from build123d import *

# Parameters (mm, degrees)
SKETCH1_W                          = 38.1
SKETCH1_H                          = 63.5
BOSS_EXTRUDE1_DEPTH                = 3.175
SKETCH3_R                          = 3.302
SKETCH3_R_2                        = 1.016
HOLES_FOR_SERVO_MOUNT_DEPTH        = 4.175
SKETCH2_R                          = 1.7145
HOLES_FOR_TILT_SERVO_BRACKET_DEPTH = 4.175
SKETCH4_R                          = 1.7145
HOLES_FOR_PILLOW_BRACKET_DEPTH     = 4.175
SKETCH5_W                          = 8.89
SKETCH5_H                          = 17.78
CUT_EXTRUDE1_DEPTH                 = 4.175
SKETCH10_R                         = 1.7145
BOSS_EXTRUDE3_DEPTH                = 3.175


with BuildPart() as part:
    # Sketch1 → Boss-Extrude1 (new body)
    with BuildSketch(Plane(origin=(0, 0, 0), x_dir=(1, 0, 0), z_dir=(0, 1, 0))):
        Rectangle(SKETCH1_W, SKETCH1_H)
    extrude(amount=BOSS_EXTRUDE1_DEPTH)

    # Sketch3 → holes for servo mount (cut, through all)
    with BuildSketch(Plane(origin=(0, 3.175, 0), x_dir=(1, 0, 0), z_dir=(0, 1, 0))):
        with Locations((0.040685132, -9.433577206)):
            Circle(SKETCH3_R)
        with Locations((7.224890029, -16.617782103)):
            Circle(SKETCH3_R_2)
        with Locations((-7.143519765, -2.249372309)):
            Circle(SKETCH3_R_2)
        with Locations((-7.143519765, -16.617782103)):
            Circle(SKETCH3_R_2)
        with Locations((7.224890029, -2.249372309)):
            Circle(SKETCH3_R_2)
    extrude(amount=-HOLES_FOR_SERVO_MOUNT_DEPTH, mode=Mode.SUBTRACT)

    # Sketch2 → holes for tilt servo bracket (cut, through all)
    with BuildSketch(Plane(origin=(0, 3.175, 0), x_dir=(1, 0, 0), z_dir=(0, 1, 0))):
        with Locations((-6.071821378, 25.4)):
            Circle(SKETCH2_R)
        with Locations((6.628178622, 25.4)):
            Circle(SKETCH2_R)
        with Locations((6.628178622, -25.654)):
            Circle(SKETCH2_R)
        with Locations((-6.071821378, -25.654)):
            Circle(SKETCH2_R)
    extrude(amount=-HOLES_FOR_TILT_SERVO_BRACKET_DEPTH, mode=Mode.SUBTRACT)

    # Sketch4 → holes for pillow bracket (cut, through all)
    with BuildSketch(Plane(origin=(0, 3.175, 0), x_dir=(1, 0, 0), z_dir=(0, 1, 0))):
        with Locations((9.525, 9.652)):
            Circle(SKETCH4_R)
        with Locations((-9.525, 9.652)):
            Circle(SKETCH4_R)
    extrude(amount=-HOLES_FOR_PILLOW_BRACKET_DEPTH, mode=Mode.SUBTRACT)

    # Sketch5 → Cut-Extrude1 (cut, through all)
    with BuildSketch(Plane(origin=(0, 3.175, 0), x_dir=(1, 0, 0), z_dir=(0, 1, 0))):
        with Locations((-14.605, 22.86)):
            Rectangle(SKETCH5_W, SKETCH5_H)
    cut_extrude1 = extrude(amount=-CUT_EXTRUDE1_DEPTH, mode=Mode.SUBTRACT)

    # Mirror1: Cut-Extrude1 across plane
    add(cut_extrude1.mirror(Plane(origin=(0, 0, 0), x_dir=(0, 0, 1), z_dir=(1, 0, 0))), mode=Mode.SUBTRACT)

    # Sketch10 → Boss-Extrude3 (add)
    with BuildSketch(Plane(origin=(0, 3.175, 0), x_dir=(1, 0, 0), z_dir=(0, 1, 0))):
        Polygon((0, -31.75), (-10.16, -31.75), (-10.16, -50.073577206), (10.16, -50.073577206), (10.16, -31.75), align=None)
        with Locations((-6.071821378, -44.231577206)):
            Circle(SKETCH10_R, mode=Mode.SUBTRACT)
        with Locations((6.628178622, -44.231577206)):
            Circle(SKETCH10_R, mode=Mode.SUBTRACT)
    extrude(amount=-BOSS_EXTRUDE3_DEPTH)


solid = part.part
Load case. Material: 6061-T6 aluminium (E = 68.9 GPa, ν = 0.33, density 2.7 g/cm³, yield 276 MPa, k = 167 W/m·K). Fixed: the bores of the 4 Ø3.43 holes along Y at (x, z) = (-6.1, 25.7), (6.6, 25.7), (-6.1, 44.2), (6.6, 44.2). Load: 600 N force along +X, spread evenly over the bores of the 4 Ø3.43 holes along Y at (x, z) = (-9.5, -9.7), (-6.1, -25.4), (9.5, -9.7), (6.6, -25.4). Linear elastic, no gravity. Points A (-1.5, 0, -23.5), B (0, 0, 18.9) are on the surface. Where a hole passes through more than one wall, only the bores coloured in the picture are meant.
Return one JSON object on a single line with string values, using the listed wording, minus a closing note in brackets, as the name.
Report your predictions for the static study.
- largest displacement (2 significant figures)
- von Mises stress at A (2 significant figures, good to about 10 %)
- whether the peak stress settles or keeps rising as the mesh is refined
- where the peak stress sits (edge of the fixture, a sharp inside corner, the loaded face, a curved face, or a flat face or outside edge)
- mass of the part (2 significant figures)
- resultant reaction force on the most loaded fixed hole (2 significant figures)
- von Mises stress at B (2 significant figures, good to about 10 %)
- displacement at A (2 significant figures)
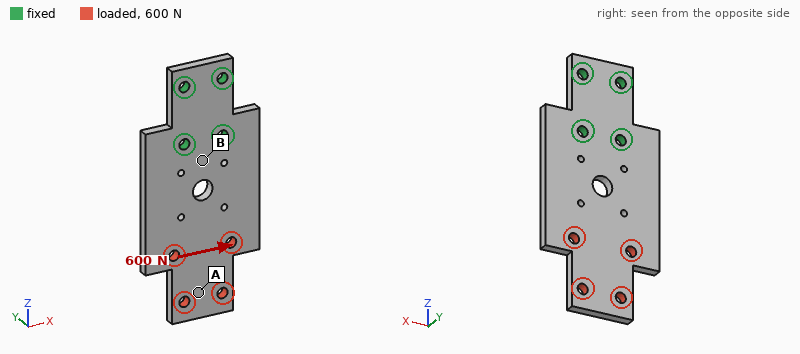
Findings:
{"largest displacement": "79 µm", "von Mises stress at A": "9.0 MPa", "whether the peak stress settles or keeps rising as the mesh is refined": "keeps rising", "where the peak stress sits": "edge of the fixture", "mass of the part": "20 g", "resultant reaction force on the most loaded fixed hole": "1.3 kN", "von Mises stress at B": "36 MPa", "displacement at A": "64 µm"}
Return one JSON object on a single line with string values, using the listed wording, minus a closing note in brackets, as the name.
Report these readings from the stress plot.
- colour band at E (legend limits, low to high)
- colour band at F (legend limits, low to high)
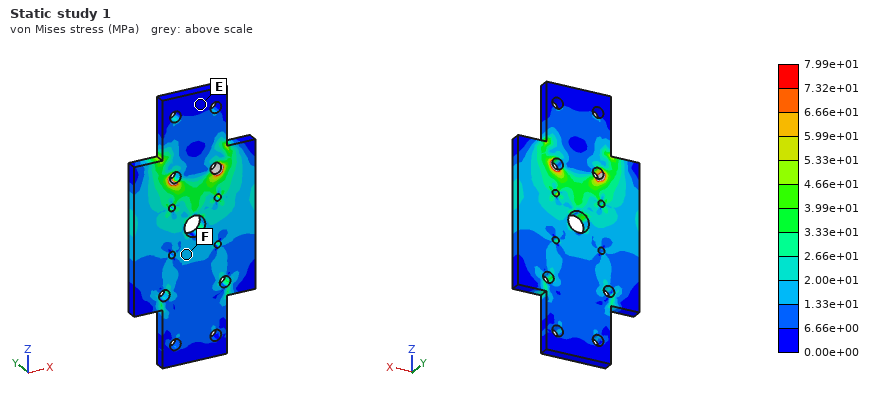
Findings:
{"colour band at E": "0.00e+00 to 6.66e+00 MPa", "colour band at F": "1.33e+01 to 2.00e+01 MPa"}
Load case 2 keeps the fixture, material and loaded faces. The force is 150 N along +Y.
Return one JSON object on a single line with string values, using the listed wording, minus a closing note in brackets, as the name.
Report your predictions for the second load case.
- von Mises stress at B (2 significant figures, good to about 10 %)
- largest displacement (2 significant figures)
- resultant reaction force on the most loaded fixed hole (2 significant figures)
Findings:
{"von Mises stress at B": "82 MPa", "largest displacement": "0.97 mm", "resultant reaction force on the most loaded fixed hole": "100 N"}
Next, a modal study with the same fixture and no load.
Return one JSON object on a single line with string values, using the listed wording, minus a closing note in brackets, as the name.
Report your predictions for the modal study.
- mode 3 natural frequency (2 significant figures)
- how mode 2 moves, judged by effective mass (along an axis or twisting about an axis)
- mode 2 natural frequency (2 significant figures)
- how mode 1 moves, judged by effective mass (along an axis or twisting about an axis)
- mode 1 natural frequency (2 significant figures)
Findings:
{"mode 3 natural frequency": "4700 Hz", "how mode 2 moves, judged by effective mass": "twisting about Z", "mode 2 natural frequency": "3300 Hz", "how mode 1 moves, judged by effective mass": "along Y", "mode 1 natural frequency": "970 Hz"}
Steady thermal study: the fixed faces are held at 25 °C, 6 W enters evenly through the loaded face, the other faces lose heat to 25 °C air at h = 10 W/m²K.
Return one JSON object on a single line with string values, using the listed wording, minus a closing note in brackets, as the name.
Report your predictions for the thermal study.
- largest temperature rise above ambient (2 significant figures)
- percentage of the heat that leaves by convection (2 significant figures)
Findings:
{"largest temperature rise above ambient": "17 K", "percentage of the heat that leaves by convection": "5.9 %"}
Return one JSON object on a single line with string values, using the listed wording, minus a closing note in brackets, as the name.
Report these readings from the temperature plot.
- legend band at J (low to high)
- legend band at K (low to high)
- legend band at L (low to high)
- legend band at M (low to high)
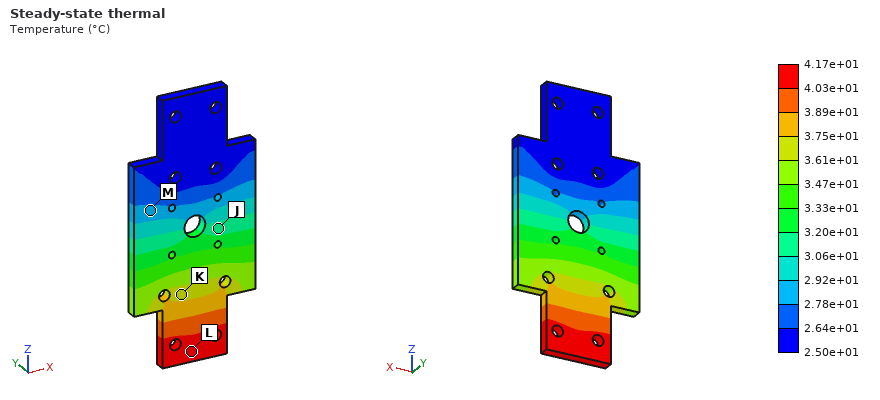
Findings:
{"legend band at J": "3.06e+01 to 3.20e+01 °C", "legend band at K": "3.61e+01 to 3.75e+01 °C", "legend band at L": "4.03e+01 to 4.17e+01 °C", "legend band at M": "2.78e+01 to 2.92e+01 °C"}
